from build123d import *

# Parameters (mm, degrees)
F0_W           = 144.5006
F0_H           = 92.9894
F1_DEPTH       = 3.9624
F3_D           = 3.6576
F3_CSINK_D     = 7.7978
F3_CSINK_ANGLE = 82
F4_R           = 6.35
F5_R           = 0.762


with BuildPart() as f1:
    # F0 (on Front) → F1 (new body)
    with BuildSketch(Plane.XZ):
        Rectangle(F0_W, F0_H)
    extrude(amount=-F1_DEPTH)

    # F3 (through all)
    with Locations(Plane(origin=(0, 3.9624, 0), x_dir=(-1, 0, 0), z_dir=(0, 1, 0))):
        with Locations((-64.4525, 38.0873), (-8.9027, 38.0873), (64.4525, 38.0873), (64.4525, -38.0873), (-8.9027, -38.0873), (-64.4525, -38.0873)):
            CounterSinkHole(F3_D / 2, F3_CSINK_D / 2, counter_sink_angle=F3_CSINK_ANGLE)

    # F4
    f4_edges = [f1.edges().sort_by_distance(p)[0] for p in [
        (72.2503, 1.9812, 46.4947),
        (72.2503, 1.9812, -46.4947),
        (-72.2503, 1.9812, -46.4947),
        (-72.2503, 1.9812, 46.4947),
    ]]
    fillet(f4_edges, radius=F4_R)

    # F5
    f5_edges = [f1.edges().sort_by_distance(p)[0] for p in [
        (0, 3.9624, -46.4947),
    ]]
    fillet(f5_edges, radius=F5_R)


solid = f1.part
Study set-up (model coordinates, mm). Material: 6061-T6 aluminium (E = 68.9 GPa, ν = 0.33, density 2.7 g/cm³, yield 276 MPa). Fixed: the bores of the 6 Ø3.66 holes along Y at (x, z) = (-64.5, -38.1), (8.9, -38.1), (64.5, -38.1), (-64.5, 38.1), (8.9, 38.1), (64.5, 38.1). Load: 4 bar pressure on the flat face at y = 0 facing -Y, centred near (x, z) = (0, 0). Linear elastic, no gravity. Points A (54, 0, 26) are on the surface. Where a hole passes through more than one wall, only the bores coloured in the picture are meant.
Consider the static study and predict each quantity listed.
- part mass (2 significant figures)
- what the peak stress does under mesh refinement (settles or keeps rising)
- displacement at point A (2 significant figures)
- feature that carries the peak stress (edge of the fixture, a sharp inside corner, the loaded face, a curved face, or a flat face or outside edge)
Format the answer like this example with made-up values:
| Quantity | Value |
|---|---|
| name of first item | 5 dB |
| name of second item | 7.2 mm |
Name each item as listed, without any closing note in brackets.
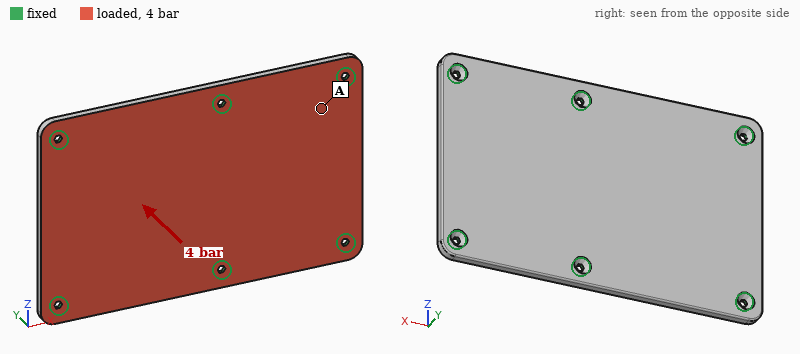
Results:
| Quantity | Value |
|---|---|
| part mass | 140 g |
| what the peak stress does under mesh refinement | keeps rising |
| displacement at point A | 0.098 mm |
| feature that carries the peak stress | edge of the fixture |
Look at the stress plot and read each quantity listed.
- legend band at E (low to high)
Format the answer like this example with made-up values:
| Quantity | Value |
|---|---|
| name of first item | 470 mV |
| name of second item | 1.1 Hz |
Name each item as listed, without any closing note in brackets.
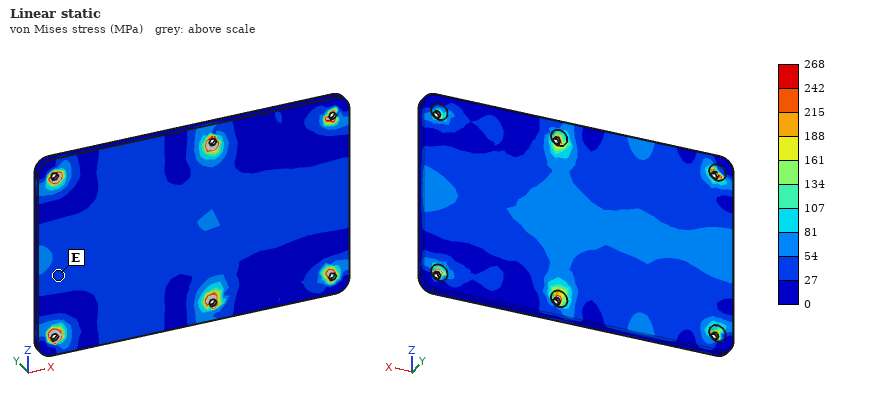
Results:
| Quantity | Value |
|---|---|
| legend band at E | 27 to 54 MPa |
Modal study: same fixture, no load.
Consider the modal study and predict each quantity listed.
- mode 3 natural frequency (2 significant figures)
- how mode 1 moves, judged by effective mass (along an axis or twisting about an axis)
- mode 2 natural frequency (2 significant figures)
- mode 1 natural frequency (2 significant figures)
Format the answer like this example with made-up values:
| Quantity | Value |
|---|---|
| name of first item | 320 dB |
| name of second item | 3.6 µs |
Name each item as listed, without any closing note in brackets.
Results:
| Quantity | Value |
|---|---|
| mode 3 natural frequency | 3500 Hz |
| how mode 1 moves, judged by effective mass | along Y |
| mode 2 natural frequency | 2600 Hz |
| mode 1 natural frequency | 2100 Hz |
